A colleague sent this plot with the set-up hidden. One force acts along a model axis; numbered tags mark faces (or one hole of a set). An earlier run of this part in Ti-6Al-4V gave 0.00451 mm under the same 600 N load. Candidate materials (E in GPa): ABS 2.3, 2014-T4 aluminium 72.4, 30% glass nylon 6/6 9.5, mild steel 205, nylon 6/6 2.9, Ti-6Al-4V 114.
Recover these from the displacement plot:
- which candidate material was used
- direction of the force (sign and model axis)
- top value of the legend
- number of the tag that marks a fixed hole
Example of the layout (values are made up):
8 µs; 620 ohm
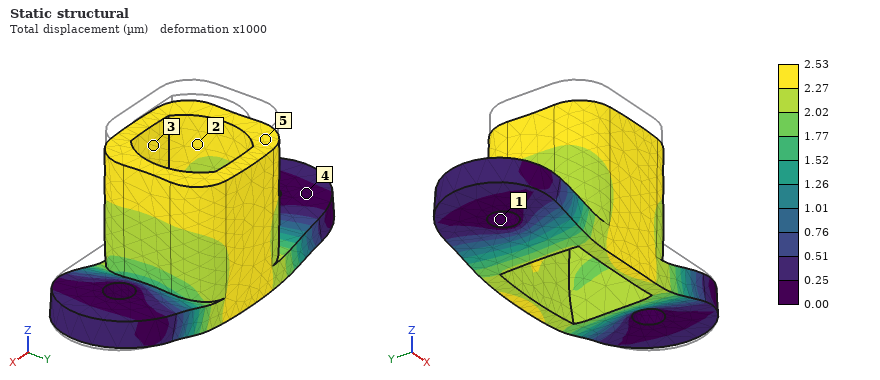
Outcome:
mild steel; -Z; 2.53 µm; 1
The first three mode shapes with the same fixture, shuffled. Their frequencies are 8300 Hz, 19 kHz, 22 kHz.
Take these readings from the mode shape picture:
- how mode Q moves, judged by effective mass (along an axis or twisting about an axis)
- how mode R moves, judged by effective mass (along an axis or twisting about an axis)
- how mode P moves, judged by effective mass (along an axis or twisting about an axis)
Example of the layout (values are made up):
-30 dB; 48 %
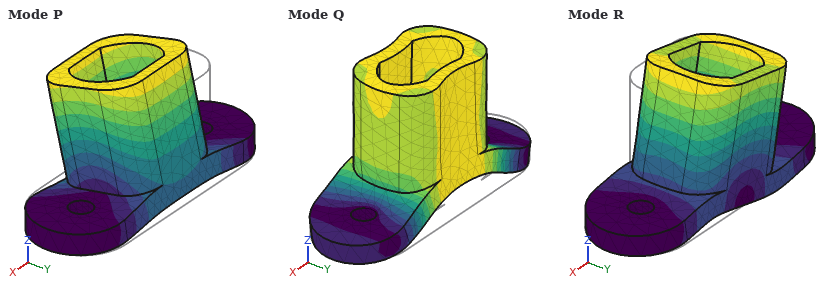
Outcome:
along Z; along X; along Y
